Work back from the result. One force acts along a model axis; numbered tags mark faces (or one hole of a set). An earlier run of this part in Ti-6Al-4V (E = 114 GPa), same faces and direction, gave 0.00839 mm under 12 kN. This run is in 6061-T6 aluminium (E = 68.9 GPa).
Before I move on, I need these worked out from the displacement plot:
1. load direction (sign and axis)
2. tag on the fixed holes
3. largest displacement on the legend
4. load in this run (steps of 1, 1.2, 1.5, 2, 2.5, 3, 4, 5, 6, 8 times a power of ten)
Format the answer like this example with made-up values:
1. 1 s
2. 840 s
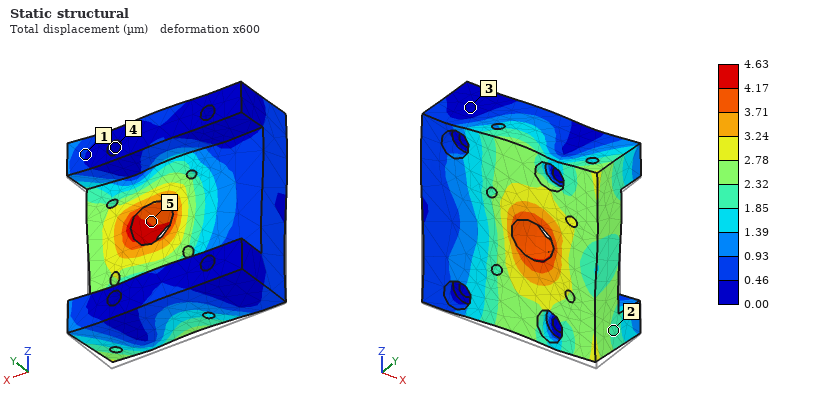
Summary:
1. +Z
2. 4
3. 4.63 µm
4. 4 kN
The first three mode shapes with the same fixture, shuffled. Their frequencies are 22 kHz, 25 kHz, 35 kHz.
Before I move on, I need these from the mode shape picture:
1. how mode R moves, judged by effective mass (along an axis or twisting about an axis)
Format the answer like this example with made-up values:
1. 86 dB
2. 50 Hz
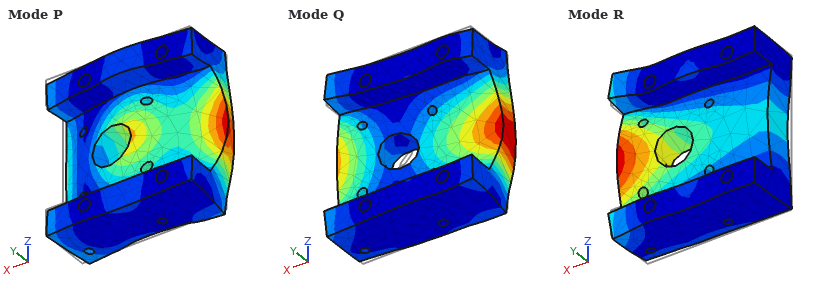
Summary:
1. along Y
